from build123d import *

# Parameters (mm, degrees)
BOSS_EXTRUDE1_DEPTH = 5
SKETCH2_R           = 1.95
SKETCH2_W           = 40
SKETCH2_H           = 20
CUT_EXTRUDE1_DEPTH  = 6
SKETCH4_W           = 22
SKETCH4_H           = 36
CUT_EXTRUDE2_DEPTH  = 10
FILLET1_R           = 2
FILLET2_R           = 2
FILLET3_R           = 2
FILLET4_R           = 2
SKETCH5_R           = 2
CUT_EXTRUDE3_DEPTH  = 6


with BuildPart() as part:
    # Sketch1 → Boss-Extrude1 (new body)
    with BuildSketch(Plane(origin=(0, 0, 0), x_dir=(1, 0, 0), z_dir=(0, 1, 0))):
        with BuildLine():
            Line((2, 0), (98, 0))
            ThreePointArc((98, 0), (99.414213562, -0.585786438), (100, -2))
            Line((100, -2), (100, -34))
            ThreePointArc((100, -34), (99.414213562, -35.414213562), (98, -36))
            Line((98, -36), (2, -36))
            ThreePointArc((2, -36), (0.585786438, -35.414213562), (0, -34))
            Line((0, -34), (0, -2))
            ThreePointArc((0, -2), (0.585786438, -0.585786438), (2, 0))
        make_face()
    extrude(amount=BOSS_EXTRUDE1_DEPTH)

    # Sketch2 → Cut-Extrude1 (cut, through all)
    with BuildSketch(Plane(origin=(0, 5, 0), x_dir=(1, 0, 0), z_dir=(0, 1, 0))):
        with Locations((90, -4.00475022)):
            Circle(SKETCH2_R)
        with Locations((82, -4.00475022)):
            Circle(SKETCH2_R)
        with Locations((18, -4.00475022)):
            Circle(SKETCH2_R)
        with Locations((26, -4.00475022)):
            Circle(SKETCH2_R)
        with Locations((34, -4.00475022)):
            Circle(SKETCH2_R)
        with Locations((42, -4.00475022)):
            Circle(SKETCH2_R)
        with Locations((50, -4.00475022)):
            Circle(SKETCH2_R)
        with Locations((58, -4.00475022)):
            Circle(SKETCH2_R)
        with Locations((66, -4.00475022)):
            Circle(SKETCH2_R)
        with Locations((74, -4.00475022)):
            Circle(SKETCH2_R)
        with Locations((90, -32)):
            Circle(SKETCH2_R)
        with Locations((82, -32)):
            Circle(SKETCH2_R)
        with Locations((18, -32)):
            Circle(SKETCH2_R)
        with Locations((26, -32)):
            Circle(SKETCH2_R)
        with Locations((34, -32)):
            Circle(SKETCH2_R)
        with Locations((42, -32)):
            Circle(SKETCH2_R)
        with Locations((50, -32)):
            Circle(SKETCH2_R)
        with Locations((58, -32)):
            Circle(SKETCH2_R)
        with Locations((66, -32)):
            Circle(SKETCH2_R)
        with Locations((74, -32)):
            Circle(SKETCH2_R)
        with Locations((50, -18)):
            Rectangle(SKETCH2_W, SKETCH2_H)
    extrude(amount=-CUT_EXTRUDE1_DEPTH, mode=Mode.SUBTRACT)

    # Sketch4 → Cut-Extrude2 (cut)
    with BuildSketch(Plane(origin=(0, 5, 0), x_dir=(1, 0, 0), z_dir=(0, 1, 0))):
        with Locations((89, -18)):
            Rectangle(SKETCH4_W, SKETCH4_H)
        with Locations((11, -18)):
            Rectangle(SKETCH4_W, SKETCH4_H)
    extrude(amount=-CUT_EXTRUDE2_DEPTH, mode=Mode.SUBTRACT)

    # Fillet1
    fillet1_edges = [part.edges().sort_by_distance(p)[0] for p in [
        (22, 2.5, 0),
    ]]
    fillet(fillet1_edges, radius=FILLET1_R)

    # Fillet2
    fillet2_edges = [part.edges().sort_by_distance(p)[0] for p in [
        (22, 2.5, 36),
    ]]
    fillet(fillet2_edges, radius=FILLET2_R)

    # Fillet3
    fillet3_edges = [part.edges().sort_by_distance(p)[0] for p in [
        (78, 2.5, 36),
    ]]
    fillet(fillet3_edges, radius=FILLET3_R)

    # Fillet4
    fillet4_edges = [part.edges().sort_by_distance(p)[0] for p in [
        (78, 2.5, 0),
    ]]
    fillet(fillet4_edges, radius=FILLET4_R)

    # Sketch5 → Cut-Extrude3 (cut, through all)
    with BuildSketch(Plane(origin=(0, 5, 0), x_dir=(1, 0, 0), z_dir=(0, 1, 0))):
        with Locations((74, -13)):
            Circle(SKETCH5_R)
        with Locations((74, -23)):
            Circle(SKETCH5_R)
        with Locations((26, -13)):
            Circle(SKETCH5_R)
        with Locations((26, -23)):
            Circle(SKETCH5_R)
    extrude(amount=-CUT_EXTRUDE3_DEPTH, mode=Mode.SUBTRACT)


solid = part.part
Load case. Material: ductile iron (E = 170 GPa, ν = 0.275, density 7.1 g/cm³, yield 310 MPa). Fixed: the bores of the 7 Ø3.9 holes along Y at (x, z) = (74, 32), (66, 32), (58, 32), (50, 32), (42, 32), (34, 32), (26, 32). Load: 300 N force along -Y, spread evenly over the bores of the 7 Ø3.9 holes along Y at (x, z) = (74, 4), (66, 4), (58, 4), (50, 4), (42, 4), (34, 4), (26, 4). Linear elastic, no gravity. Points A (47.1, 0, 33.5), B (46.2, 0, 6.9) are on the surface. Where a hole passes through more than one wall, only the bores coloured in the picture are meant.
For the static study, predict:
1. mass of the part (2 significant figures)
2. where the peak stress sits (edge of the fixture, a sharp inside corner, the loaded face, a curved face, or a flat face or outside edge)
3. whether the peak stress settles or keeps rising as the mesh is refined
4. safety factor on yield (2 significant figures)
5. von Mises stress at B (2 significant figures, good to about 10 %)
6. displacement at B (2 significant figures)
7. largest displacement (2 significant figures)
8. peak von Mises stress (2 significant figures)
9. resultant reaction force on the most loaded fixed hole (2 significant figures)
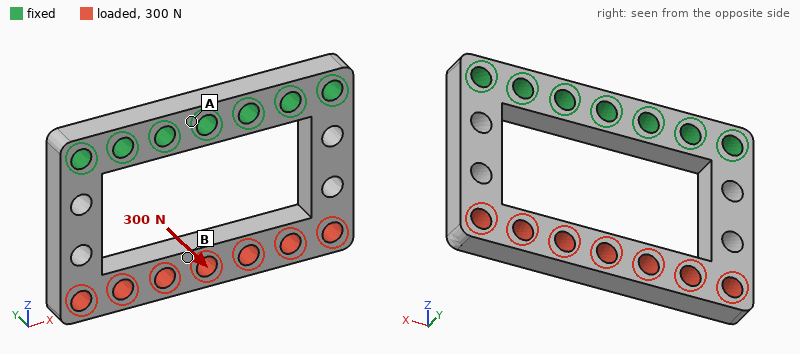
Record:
35 g
a curved face
settles
1.2
36 MPa
0.10 mm
0.14 mm
260 MPa
120 N
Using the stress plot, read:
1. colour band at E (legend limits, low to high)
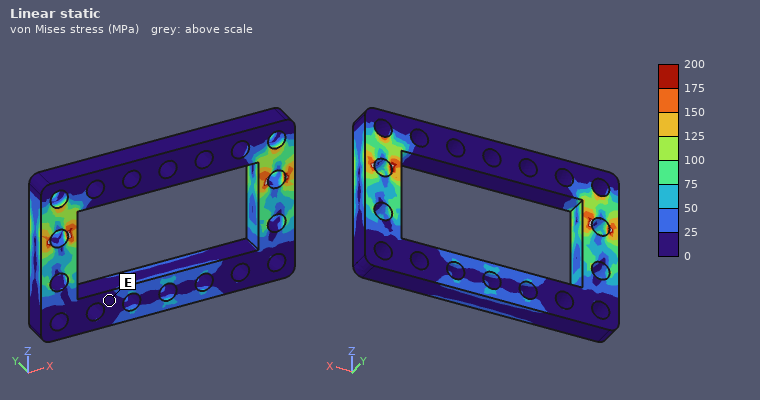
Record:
0 to 25 MPa
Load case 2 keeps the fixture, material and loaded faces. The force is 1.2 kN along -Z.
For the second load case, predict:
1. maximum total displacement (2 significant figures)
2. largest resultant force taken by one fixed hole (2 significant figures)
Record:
25 µm
630 N
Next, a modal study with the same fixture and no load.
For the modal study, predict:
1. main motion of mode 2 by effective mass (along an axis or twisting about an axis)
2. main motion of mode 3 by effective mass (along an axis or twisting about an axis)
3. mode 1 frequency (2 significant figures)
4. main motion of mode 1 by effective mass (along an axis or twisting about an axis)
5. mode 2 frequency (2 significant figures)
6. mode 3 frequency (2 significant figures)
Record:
twisting about Z
along X
2200 Hz
along Y
4400 Hz
5600 Hz
